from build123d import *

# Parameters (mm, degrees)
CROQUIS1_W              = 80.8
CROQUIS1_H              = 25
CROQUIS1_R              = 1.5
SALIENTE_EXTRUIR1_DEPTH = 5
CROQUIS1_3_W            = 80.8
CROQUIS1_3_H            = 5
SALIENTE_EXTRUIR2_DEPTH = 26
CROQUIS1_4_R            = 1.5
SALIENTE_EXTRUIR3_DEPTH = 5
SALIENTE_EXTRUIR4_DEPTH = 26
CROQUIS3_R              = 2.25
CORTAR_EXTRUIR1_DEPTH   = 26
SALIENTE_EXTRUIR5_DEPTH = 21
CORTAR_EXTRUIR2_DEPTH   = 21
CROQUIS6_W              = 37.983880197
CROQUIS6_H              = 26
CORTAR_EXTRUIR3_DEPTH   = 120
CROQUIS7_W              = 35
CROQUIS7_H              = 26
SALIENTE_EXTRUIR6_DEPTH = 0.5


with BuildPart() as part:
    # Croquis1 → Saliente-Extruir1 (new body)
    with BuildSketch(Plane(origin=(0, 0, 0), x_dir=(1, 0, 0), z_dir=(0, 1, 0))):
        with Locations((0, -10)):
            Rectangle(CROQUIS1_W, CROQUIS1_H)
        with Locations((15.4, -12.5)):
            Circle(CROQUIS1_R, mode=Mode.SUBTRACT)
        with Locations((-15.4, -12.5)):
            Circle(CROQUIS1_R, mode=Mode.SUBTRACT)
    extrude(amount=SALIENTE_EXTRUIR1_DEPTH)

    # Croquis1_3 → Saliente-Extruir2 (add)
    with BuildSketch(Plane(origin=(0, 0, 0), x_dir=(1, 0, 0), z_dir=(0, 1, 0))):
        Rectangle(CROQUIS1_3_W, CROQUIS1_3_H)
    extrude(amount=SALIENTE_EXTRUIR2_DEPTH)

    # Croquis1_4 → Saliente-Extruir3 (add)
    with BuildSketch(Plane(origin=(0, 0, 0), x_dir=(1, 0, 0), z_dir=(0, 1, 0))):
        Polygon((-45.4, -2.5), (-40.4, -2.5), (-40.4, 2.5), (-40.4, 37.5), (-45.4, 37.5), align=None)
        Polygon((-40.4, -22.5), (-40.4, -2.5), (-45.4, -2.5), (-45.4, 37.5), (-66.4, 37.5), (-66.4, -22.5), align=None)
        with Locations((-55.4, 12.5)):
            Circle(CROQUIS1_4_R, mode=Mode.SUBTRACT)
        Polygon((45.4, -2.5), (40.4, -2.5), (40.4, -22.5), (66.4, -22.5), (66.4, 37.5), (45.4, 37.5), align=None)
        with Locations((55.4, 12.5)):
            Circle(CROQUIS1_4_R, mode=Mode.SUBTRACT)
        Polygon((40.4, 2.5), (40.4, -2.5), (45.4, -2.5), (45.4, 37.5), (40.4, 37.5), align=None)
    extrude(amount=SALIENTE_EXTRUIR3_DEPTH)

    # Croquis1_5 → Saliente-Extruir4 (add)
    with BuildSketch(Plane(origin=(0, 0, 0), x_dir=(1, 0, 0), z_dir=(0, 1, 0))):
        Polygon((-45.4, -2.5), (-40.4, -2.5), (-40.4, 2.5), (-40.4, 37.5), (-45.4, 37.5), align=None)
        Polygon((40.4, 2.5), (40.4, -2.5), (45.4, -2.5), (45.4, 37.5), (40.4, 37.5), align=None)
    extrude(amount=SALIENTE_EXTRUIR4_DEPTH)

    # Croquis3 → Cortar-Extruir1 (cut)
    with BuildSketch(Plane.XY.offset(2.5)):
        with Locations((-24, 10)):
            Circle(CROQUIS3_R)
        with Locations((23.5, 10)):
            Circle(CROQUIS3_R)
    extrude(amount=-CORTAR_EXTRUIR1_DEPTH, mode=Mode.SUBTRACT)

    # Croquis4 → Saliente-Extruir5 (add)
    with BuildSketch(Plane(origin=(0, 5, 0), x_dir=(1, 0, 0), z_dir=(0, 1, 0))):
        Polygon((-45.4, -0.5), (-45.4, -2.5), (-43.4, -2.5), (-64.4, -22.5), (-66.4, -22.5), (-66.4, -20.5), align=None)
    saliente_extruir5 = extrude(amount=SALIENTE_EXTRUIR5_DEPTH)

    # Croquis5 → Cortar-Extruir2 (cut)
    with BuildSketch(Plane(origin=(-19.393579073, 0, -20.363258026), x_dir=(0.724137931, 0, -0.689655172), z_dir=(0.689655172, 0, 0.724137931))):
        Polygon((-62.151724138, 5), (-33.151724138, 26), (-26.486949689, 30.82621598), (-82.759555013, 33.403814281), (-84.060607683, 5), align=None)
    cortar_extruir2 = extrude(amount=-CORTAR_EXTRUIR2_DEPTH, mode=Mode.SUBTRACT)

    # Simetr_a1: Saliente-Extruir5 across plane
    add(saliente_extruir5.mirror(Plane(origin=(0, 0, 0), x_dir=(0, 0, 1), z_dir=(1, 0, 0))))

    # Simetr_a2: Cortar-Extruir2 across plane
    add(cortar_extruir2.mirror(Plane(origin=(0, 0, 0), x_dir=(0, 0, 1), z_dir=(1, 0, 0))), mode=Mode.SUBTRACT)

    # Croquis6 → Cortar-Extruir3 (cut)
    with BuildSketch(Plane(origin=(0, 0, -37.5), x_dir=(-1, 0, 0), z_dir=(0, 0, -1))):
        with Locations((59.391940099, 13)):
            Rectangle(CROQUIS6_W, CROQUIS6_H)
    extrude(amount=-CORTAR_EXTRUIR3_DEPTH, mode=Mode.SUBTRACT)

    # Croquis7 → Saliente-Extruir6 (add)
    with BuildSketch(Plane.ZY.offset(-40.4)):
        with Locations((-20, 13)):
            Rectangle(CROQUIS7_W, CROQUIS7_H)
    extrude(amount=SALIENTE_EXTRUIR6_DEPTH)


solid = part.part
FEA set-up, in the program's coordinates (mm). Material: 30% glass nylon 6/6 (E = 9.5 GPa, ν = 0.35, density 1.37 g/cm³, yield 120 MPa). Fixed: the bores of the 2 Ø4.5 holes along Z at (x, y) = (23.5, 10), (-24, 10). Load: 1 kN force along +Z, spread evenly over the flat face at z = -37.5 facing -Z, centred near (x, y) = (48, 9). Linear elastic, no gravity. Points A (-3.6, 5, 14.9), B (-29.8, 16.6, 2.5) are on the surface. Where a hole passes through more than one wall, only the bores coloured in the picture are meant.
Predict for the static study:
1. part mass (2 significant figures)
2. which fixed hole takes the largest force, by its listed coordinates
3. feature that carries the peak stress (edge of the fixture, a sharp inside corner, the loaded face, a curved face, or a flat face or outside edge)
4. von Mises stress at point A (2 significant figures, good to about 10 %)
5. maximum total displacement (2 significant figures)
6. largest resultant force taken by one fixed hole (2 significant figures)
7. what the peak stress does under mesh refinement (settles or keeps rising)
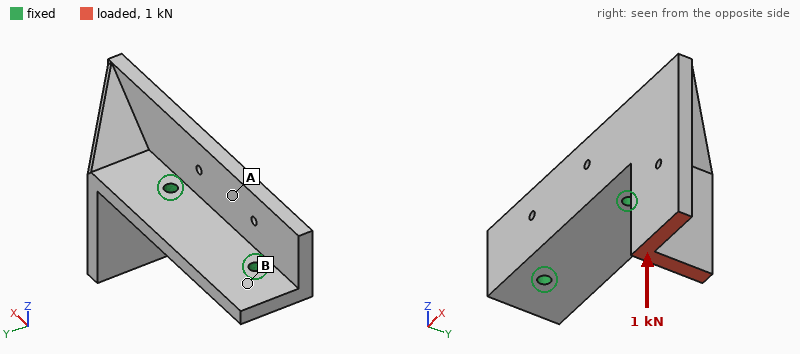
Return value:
43 g
(23.5, 10)
edge of the fixture
12 MPa
0.69 mm
1.5 kN
keeps rising
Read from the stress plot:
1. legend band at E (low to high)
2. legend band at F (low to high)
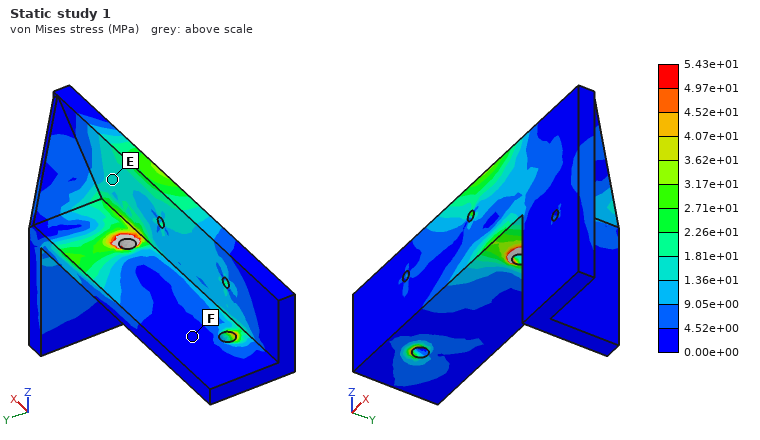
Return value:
1.36e+01 to 1.81e+01 MPa
0.00e+00 to 4.52e+00 MPa
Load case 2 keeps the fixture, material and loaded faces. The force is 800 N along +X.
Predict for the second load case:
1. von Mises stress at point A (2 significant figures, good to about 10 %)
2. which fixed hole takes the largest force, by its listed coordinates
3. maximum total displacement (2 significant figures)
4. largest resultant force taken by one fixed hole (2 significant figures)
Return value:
16 MPa
(23.5, 10)
1.5 mm
1.5 kN
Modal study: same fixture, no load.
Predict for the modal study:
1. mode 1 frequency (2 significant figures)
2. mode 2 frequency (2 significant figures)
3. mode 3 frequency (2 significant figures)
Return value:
1000 Hz
1400 Hz
2100 Hz
